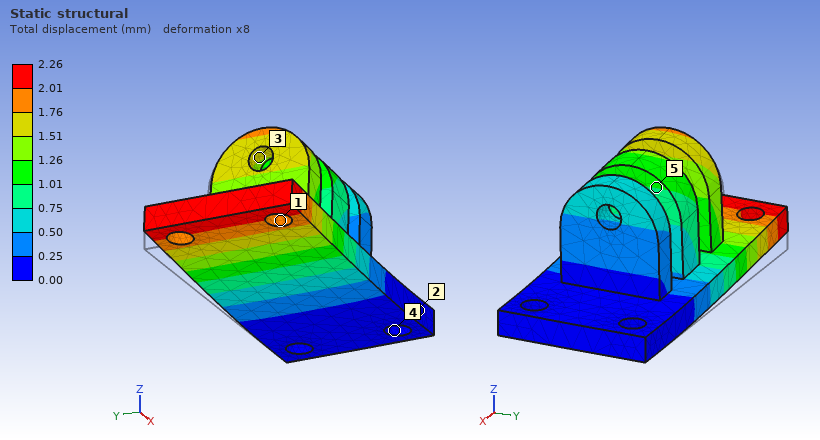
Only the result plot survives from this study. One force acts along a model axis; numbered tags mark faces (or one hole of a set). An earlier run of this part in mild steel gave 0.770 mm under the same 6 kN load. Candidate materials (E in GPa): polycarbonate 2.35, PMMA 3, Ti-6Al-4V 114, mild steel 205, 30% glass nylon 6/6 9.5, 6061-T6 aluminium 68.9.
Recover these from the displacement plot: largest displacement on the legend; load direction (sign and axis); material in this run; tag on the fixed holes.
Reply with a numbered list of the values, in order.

1. 2.26 mm
2. +Z
3. 6061-T6 aluminium
4. 4
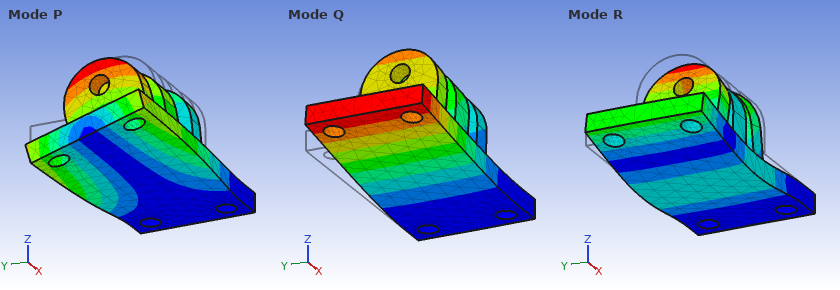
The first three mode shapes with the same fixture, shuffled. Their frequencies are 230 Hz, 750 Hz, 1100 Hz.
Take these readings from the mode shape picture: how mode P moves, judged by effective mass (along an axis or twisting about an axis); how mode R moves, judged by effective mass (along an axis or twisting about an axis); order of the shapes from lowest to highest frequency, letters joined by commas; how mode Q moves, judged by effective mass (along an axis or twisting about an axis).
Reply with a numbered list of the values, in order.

1. along Y
2. along Z
3. Q, P, R
4. along Z
